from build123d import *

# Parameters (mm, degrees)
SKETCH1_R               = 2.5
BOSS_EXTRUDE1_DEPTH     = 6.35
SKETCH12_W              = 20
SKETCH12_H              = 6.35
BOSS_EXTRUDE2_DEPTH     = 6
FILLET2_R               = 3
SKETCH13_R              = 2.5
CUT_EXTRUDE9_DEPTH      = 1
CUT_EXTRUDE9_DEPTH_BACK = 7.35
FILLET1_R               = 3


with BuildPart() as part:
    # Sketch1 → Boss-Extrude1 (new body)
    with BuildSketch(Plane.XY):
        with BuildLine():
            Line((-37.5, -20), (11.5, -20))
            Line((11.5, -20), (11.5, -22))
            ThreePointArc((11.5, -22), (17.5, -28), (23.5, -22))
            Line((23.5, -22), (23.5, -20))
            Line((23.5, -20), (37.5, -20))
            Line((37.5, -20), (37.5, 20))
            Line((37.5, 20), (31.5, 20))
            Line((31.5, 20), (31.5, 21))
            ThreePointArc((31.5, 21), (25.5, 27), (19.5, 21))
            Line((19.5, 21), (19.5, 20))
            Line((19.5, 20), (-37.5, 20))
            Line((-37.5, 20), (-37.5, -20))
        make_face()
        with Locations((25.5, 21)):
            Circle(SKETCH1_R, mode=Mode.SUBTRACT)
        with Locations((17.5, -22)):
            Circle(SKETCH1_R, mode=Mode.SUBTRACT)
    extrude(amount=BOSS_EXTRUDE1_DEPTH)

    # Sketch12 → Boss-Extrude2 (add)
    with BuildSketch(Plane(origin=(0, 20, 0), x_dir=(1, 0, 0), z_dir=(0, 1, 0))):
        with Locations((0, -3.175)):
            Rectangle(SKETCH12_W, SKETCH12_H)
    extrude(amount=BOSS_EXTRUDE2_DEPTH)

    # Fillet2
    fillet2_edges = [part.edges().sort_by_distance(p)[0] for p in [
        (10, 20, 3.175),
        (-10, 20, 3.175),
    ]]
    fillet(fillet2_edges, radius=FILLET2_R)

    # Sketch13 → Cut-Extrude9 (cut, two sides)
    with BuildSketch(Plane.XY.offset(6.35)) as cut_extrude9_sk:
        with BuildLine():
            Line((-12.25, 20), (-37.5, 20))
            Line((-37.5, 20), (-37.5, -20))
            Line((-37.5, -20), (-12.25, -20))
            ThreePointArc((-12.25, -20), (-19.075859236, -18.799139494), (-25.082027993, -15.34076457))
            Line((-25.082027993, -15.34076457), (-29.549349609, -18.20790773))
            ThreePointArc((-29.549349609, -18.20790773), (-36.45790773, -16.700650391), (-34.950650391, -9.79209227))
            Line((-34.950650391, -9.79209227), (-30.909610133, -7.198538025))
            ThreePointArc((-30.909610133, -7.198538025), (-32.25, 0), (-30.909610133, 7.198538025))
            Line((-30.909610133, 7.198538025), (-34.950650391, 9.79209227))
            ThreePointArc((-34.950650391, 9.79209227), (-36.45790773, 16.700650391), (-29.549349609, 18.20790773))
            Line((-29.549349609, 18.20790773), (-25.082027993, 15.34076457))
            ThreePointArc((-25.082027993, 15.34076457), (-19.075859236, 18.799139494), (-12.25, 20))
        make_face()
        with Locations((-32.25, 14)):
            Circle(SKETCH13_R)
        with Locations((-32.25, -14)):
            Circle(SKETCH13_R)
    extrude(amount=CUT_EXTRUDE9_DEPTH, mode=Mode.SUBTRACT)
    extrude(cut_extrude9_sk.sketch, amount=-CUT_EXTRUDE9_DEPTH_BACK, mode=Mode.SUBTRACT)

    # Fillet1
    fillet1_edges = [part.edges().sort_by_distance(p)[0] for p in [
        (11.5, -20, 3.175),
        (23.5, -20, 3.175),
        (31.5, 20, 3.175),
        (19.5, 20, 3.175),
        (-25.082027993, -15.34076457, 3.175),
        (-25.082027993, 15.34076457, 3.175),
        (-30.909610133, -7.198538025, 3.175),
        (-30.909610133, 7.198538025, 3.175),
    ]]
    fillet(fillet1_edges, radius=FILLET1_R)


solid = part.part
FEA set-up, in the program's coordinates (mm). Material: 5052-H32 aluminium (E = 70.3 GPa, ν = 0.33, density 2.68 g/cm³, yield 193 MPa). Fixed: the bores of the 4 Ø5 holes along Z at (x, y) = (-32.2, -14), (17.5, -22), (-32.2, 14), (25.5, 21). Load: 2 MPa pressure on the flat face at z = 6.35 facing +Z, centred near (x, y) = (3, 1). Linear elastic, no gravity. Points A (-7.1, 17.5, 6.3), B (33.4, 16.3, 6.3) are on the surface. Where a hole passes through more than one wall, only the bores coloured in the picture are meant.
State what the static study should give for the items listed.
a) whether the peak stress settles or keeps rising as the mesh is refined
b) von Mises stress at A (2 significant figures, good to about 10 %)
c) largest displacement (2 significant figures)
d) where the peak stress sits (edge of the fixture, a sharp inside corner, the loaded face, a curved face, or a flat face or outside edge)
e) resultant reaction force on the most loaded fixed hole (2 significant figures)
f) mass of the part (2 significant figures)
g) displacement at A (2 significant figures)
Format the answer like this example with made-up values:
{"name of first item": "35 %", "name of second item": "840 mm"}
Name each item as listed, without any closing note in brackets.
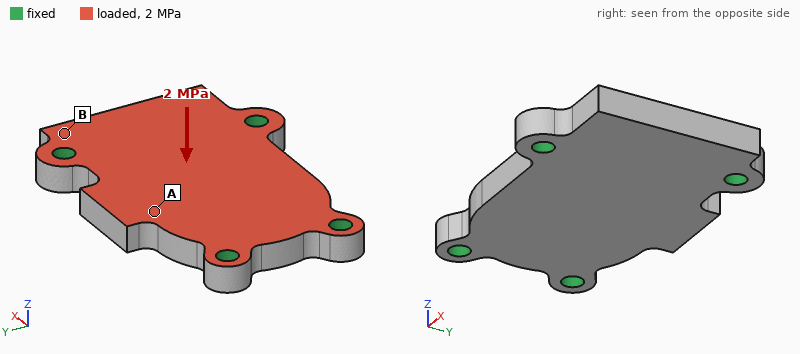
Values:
{"whether the peak stress settles or keeps rising as the mesh is refined": "keeps rising", "von Mises stress at A": "49 MPa", "largest displacement": "69 µm", "where the peak stress sits": "edge of the fixture", "resultant reaction force on the most loaded fixed hole": "1.9 kN", "mass of the part": "51 g", "displacement at A": "58 µm"}
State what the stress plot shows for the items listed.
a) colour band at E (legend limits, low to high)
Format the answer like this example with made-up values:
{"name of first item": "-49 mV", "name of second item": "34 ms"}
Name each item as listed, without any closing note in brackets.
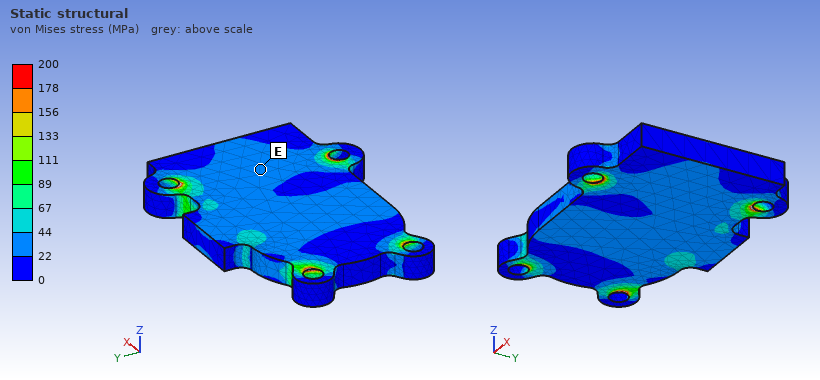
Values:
{"colour band at E": "22 to 44 MPa"}
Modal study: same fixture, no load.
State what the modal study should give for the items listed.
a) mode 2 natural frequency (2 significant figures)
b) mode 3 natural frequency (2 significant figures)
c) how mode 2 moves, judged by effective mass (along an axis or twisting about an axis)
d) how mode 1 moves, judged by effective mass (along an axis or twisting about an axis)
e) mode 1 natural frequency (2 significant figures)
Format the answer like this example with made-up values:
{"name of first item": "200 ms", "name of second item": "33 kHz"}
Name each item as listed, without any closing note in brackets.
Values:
{"mode 2 natural frequency": "11 kHz", "mode 3 natural frequency": "12 kHz", "how mode 2 moves, judged by effective mass": "along Z", "how mode 1 moves, judged by effective mass": "along Z", "mode 1 natural frequency": "8100 Hz"}
